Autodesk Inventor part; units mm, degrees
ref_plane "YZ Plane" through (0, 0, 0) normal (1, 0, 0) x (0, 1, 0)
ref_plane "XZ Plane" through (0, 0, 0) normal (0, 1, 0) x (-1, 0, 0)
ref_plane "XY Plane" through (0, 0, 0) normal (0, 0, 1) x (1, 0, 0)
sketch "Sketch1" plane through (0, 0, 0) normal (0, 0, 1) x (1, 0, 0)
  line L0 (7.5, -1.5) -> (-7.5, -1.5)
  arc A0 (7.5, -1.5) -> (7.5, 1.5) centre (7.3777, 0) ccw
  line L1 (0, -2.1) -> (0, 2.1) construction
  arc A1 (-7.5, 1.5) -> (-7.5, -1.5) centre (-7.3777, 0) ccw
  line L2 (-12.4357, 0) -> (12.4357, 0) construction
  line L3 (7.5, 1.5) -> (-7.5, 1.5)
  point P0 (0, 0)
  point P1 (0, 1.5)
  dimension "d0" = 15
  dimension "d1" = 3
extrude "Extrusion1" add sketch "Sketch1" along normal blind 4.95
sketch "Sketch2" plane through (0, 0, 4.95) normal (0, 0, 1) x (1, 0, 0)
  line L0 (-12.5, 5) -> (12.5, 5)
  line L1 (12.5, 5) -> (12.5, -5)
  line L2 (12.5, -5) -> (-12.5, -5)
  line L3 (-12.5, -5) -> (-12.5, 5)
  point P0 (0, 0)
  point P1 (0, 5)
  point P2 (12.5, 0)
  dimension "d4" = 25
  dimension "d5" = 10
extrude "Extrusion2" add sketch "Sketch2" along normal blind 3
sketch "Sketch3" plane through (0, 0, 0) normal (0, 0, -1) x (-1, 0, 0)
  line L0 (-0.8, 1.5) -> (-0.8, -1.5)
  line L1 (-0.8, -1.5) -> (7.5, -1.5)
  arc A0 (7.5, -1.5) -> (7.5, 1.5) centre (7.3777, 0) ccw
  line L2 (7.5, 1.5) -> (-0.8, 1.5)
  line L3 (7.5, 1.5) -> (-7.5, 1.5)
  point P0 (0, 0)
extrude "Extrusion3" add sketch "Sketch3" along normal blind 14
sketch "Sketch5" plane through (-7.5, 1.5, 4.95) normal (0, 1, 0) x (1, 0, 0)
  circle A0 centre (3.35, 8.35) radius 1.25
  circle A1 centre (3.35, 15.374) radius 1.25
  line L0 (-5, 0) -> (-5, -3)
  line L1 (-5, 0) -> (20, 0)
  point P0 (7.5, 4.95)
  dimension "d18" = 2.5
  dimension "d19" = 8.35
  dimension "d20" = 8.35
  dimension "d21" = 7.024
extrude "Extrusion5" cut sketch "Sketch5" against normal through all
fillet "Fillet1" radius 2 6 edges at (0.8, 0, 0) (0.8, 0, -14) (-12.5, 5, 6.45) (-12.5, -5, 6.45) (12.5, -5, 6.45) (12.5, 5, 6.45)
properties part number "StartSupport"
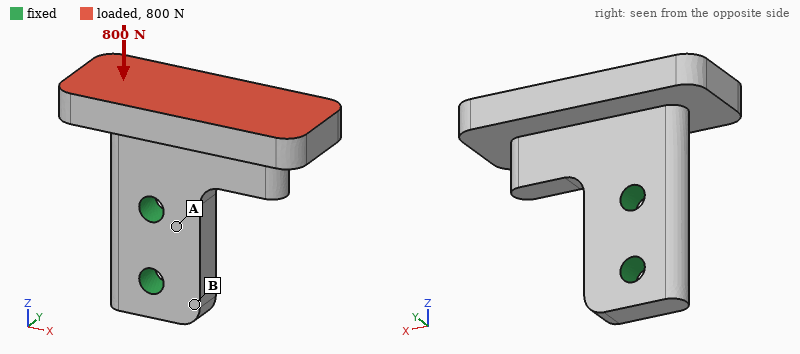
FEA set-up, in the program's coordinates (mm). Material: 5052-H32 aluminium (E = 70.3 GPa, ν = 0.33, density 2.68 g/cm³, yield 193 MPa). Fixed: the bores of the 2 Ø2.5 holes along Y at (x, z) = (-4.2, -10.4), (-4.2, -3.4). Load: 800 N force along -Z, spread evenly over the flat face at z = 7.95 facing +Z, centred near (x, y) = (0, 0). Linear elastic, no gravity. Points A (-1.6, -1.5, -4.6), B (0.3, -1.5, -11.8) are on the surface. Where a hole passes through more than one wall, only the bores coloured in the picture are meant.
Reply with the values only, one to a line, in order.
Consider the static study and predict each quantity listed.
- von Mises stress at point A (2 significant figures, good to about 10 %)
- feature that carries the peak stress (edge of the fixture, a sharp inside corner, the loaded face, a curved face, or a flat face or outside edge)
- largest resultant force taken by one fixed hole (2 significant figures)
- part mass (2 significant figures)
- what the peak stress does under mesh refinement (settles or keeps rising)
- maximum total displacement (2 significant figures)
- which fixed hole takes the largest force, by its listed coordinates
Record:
51 MPa
edge of the fixture
690 N
3.6 g
keeps rising
54 µm
(-4.2, -3.4)
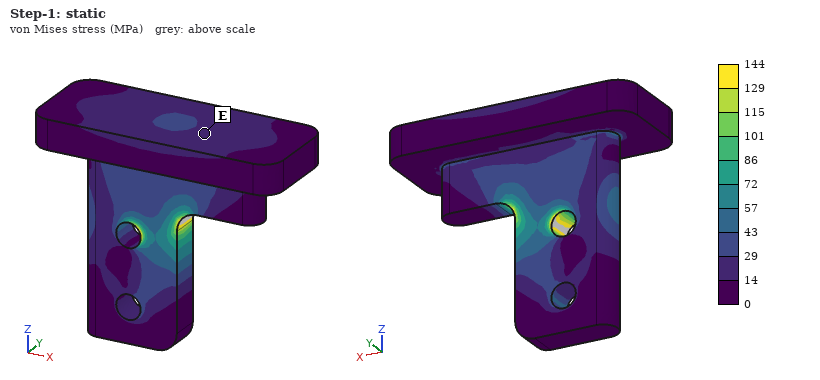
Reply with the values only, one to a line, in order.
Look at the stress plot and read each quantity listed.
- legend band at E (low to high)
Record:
14 to 29 MPa
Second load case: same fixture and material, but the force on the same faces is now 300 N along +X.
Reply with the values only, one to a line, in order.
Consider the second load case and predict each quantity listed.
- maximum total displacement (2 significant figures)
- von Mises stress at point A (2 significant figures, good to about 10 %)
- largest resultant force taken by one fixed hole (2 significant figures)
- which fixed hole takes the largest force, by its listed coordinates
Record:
41 µm
35 MPa
560 N
(-4.2, -3.4)
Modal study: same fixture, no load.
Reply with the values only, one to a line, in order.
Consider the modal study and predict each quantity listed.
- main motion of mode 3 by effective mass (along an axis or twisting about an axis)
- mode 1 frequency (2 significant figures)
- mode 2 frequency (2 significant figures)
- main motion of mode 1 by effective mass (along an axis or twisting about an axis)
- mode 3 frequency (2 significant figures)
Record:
along X
5700 Hz
9200 Hz
along Y
11 kHz
